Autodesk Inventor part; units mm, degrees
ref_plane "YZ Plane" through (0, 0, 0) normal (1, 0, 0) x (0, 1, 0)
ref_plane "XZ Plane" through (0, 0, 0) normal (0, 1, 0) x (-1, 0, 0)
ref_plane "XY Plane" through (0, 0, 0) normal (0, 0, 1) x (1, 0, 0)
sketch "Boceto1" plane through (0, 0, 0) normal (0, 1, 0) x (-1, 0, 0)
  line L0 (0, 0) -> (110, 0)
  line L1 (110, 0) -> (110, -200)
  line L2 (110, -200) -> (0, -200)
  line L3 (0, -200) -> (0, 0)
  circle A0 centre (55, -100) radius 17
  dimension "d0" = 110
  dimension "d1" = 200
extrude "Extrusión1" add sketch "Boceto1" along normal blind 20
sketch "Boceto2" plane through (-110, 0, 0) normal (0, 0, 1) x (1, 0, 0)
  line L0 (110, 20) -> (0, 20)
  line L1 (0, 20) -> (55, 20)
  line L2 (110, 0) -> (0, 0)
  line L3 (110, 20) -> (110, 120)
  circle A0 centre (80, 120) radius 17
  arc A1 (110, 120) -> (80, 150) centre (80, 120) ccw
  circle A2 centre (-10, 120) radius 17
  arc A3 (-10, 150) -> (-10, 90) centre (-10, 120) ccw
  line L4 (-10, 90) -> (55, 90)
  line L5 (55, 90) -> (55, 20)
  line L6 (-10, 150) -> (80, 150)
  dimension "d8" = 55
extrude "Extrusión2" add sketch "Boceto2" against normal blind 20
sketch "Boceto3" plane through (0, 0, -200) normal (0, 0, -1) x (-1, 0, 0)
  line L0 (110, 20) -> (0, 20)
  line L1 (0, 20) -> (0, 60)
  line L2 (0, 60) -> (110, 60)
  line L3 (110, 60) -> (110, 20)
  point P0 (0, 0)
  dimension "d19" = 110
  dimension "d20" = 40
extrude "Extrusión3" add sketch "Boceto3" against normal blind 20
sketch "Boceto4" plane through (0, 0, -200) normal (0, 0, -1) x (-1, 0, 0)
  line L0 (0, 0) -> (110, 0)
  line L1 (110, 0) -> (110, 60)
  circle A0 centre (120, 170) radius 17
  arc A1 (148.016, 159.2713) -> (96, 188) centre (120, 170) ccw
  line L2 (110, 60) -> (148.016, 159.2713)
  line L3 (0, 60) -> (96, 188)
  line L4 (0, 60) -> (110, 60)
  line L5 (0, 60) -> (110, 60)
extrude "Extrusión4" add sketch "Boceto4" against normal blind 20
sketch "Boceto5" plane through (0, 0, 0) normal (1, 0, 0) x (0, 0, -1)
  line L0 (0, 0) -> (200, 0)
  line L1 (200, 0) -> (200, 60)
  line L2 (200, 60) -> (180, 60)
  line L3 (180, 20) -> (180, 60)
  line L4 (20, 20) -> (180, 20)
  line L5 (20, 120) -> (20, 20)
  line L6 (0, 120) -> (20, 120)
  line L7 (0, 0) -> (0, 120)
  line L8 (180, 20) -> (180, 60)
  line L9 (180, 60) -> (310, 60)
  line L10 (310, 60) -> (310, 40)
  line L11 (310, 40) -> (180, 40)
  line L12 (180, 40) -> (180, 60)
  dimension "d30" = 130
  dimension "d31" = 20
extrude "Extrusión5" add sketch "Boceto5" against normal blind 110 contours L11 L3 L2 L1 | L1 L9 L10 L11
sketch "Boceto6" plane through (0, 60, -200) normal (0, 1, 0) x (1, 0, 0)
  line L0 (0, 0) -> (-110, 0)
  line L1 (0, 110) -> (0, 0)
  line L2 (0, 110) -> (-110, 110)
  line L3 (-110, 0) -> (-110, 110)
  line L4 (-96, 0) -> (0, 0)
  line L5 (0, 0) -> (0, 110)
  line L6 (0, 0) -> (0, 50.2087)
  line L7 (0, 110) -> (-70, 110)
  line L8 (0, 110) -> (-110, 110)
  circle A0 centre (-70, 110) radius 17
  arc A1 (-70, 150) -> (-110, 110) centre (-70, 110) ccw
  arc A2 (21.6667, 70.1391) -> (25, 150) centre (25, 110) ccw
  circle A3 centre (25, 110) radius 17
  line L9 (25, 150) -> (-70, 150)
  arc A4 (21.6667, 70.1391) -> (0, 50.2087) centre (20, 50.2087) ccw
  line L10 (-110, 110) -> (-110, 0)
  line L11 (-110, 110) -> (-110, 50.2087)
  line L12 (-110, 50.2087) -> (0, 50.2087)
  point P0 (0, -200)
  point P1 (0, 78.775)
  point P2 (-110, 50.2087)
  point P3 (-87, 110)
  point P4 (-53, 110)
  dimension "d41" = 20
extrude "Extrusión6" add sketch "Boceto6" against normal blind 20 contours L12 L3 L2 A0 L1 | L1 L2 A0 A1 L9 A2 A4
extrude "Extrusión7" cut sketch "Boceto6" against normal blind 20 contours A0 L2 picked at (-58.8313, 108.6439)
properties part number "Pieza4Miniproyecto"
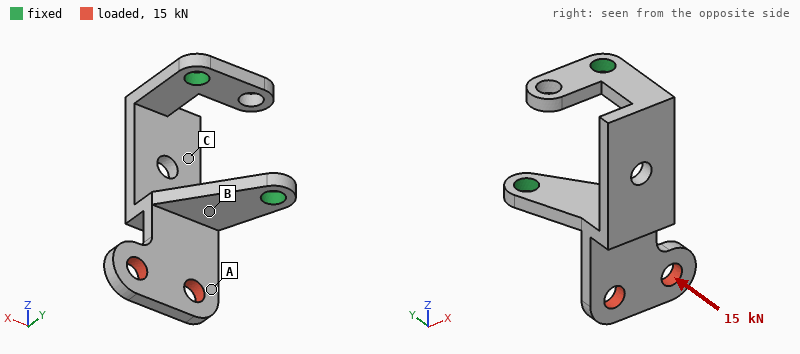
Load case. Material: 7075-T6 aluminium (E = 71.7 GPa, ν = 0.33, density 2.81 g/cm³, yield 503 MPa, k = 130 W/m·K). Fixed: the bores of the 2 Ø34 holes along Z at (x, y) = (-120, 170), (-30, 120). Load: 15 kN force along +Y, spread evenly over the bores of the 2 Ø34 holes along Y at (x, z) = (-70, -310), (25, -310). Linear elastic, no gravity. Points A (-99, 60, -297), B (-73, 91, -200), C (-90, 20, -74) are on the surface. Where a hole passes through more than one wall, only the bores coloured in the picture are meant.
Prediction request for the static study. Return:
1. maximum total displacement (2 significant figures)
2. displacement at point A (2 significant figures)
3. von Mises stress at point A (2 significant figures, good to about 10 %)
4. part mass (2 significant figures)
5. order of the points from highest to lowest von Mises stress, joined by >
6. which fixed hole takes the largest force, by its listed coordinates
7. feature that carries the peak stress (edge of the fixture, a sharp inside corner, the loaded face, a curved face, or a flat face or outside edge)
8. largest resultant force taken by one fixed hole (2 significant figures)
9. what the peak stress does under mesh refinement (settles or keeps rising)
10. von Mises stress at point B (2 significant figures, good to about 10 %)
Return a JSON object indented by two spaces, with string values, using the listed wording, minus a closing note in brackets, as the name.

{
  "maximum total displacement": "5.0 mm",
  "displacement at point A": "2.1 mm",
  "von Mises stress at point A": "55 MPa",
  "part mass": "3.7 kg",
  "order of the points from highest to lowest von Mises stress, joined by >": "B > A > C",
  "which fixed hole takes the largest force, by its listed coordinates": "(-120, 170)",
  "feature that carries the peak stress": "edge of the fixture",
  "largest resultant force taken by one fixed hole": "22 kN",
  "what the peak stress does under mesh refinement": "keeps rising",
  "von Mises stress at point B": "120 MPa"
}
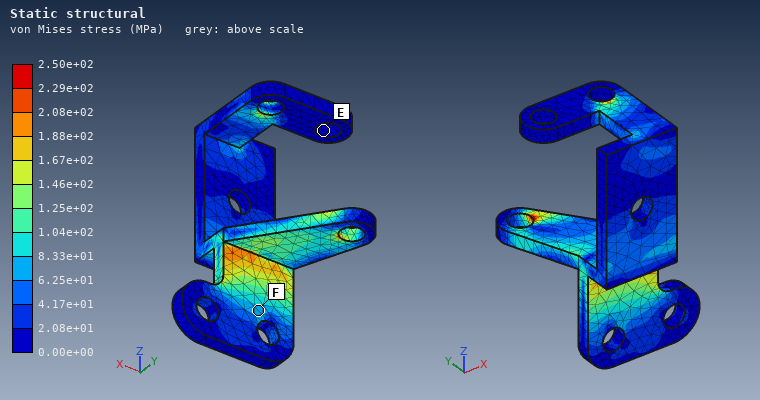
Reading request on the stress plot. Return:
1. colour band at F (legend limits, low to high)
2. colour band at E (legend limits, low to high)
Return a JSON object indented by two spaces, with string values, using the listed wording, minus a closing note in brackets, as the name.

{
  "colour band at F": "6.25e+01 to 8.33e+01 MPa",
  "colour band at E": "0.00e+00 to 2.08e+01 MPa"
}
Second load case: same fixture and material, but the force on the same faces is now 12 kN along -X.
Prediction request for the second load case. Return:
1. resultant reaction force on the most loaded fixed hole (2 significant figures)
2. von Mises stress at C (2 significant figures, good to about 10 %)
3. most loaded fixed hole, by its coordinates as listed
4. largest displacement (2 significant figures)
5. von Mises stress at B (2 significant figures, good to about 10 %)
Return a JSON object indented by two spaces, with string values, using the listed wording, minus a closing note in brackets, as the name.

{
  "resultant reaction force on the most loaded fixed hole": "17 kN",
  "von Mises stress at C": "17 MPa",
  "most loaded fixed hole, by its coordinates as listed": "(-120, 170)",
  "largest displacement": "1.8 mm",
  "von Mises stress at B": "68 MPa"
}
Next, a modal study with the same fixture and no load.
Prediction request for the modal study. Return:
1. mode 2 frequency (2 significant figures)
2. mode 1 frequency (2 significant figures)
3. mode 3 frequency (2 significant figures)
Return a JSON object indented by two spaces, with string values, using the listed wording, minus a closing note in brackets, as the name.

{
  "mode 2 frequency": "530 Hz",
  "mode 1 frequency": "370 Hz",
  "mode 3 frequency": "670 Hz"
}
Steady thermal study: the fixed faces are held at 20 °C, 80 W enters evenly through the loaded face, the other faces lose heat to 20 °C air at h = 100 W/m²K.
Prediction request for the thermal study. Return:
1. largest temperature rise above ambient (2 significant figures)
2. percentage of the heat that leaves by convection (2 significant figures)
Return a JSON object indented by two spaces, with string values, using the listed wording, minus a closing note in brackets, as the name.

{
  "largest temperature rise above ambient": "20 K",
  "percentage of the heat that leaves by convection": "92 %"
}
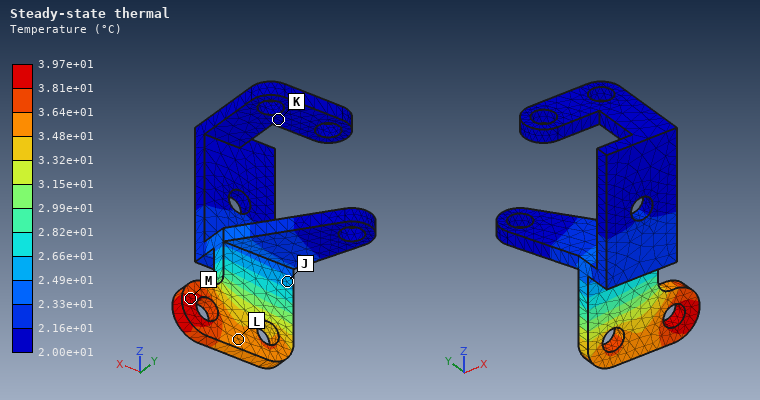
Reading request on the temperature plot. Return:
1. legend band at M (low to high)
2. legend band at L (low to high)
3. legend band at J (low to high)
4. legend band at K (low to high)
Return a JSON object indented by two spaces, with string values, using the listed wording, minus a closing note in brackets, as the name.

{
  "legend band at M": "3.81e+01 to 3.97e+01 °C",
  "legend band at L": "3.48e+01 to 3.64e+01 °C",
  "legend band at J": "2.49e+01 to 2.66e+01 °C",
  "legend band at K": "2.00e+01 to 2.16e+01 °C"
}
